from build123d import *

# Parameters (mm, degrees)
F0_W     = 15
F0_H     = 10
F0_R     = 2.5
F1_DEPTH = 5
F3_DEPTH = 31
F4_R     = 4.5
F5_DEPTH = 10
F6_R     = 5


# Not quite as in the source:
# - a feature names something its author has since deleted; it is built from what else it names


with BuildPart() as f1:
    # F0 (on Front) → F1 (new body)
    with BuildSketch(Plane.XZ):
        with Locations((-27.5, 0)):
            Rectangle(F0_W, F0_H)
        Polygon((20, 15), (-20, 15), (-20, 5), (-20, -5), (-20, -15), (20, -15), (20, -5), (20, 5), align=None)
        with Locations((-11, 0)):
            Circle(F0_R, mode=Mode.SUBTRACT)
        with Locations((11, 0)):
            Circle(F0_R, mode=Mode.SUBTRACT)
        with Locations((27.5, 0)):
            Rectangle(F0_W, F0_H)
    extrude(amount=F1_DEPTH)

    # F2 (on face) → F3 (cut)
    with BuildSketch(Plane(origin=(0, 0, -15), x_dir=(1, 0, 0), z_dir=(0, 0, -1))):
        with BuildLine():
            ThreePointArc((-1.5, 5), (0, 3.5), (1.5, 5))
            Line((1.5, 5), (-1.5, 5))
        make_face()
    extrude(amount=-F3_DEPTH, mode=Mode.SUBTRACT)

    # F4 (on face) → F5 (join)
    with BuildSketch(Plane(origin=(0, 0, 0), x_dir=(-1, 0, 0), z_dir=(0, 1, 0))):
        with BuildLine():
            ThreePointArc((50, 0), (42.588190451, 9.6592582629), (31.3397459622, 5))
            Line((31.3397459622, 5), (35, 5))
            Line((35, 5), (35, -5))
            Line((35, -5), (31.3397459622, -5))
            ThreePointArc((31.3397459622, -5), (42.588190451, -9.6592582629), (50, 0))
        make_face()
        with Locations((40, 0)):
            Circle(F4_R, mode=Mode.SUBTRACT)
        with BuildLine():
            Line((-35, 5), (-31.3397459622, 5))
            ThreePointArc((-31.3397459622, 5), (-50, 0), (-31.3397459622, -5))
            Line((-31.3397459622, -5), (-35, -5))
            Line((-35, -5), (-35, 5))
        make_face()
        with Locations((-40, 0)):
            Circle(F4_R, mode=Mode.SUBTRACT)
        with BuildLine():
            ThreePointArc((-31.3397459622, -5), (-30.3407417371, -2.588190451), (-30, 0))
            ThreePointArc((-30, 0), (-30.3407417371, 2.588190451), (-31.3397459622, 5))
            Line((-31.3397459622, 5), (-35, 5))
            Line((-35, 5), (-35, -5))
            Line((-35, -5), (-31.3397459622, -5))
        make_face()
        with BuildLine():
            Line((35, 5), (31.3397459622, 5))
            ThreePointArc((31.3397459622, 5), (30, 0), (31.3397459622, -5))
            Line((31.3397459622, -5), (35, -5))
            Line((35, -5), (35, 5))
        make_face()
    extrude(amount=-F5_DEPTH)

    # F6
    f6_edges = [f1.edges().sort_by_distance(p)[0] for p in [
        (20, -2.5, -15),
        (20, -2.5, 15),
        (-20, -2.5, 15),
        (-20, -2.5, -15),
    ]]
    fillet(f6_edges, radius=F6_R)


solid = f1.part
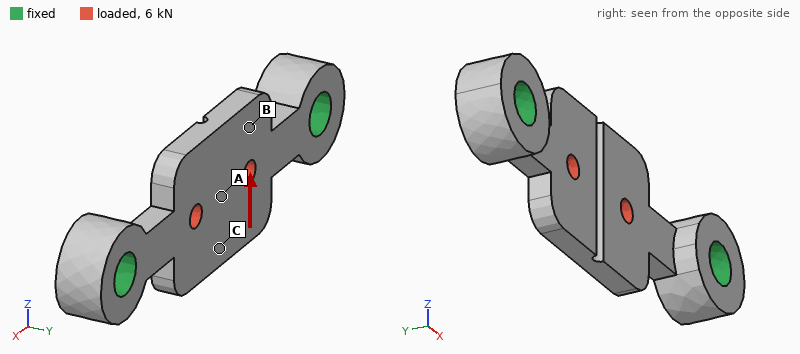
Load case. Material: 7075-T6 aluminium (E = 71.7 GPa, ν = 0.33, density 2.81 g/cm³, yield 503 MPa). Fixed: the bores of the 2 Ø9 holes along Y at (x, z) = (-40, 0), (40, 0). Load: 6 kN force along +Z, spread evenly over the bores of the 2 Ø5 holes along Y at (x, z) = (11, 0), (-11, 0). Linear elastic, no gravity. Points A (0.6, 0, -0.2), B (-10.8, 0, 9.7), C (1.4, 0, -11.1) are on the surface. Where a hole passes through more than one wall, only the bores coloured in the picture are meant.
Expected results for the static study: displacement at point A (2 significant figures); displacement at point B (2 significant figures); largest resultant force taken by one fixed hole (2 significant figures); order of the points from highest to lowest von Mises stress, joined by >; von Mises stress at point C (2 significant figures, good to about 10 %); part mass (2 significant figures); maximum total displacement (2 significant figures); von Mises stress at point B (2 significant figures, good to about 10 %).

99 µm
92 µm
3.0 kN
B > C > A
35 MPa
33 g
99 µm
57 MPa
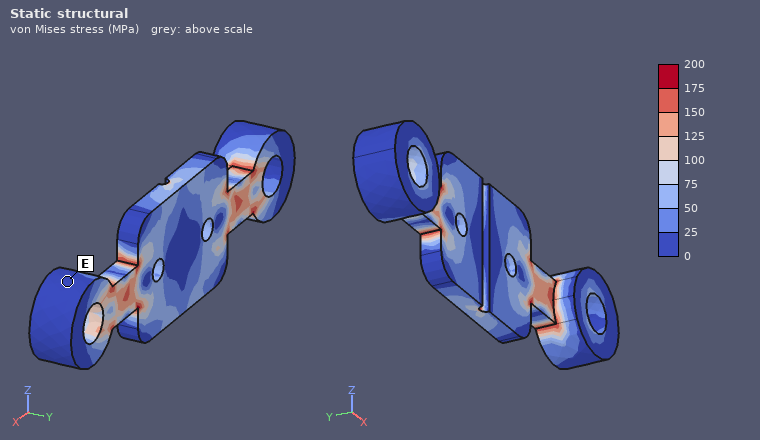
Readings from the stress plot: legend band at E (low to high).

0 to 25 MPa
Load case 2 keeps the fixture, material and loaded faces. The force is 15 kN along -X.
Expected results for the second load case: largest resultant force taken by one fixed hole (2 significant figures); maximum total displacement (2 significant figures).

7.5 kN
56 µm
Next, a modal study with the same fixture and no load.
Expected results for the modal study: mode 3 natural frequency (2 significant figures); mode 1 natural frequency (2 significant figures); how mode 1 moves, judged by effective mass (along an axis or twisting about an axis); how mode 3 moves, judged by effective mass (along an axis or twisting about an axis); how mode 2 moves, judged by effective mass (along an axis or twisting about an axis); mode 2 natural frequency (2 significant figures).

10000 Hz
4100 Hz
along Y
along Z
twisting about X
4600 Hz
